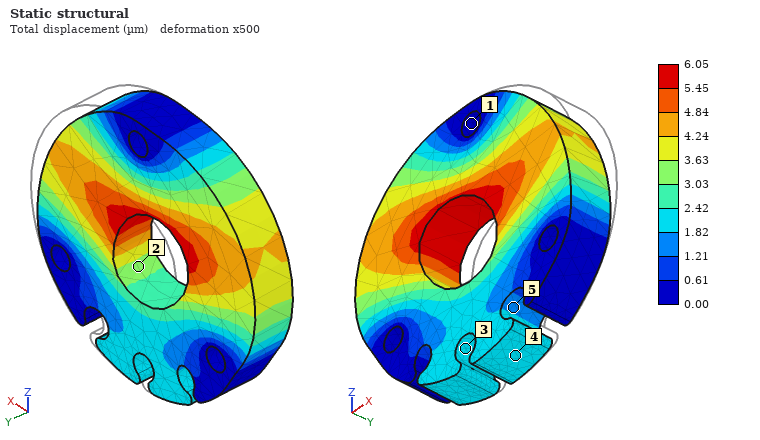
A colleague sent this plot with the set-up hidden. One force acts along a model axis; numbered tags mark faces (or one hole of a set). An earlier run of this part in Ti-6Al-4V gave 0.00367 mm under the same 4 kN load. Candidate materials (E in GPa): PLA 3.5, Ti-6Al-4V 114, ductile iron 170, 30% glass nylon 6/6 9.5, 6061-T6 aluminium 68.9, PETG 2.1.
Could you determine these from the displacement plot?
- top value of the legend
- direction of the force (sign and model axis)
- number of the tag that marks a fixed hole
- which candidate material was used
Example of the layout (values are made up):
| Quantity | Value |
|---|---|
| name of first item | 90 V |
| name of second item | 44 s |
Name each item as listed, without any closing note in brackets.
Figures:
| Quantity | Value |
|---|---|
| top value of the legend | 6.05 µm |
| direction of the force | -X |
| number of the tag that marks a fixed hole | 1 |
| which candidate material was used | 6061-T6 aluminium |
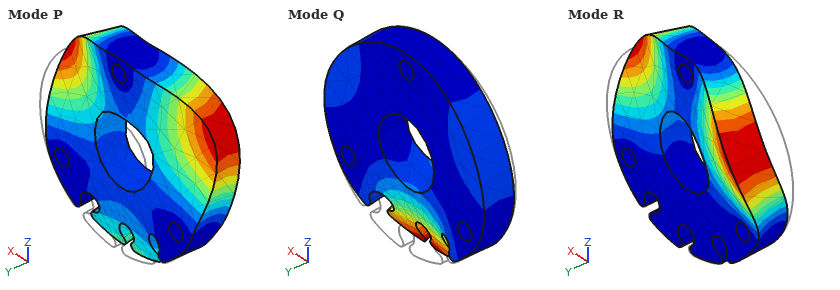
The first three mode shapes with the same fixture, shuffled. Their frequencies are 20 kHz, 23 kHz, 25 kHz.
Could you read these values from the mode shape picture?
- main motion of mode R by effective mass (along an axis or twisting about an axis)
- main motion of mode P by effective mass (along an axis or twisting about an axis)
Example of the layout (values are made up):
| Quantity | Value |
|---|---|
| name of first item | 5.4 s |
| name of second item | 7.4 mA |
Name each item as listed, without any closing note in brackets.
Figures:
| Quantity | Value |
|---|---|
| main motion of mode R by effective mass | twisting about Z |
| main motion of mode P by effective mass | along Y |
